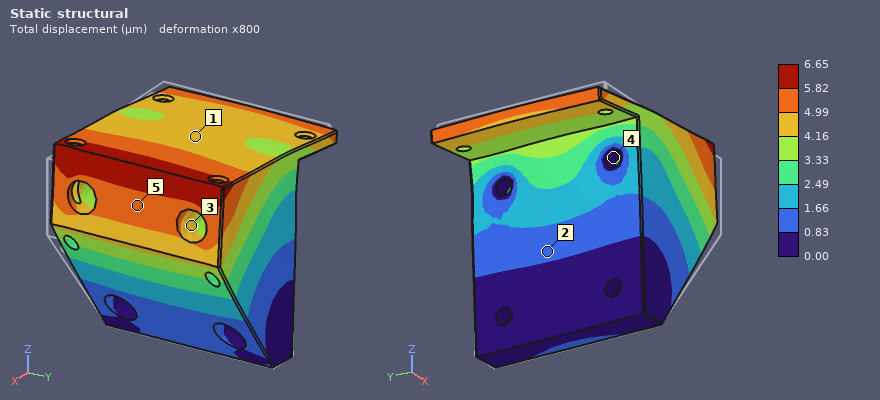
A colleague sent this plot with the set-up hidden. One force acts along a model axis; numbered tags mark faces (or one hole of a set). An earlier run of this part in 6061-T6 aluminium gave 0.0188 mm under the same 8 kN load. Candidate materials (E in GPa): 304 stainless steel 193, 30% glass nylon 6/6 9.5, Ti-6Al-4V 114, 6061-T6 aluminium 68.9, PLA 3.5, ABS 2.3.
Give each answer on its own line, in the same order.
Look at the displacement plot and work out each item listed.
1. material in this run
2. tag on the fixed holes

304 stainless steel
4
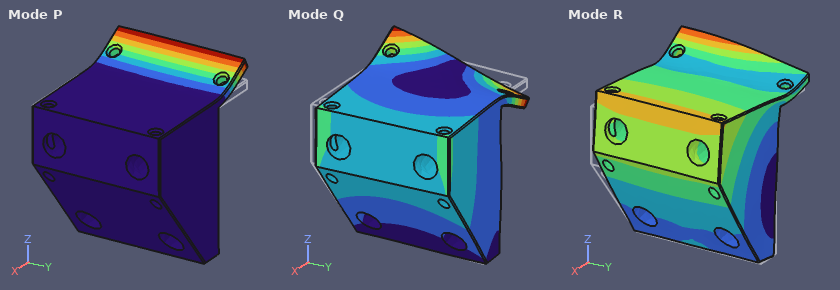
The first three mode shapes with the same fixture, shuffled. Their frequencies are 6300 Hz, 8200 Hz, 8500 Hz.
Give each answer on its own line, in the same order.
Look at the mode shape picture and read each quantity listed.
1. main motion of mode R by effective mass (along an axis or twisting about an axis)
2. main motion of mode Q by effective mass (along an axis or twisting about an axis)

along Z
along Y
